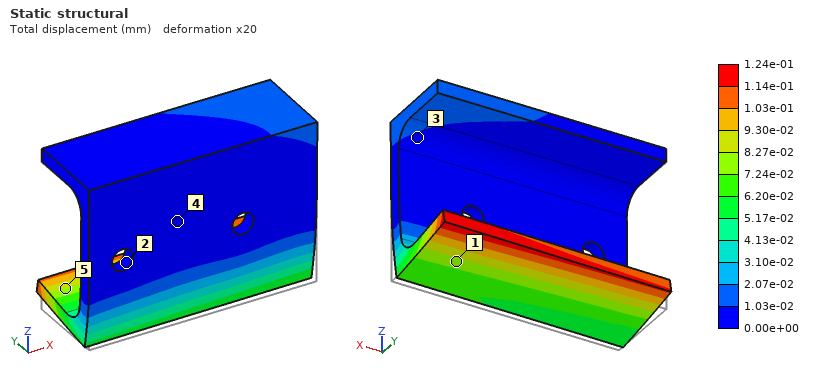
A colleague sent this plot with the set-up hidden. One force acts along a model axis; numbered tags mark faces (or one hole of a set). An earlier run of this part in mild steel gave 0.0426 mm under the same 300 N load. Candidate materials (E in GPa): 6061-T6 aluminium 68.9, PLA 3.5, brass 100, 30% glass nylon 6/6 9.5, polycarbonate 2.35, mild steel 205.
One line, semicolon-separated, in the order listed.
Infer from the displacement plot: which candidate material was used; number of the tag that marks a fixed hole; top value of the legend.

6061-T6 aluminium; 2; 1.24e-01 mm
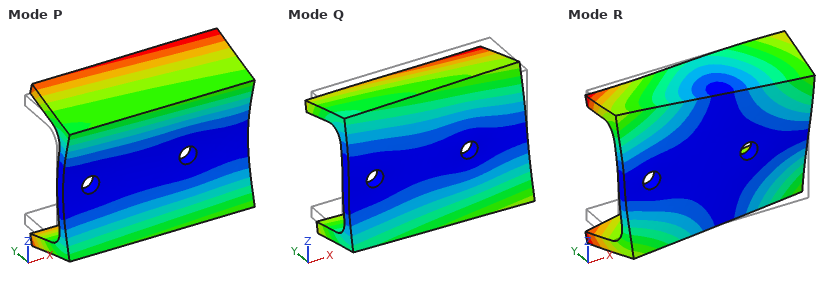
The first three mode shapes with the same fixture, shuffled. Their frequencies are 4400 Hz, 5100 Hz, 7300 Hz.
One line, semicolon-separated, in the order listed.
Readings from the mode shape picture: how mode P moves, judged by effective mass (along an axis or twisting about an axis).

along Y
